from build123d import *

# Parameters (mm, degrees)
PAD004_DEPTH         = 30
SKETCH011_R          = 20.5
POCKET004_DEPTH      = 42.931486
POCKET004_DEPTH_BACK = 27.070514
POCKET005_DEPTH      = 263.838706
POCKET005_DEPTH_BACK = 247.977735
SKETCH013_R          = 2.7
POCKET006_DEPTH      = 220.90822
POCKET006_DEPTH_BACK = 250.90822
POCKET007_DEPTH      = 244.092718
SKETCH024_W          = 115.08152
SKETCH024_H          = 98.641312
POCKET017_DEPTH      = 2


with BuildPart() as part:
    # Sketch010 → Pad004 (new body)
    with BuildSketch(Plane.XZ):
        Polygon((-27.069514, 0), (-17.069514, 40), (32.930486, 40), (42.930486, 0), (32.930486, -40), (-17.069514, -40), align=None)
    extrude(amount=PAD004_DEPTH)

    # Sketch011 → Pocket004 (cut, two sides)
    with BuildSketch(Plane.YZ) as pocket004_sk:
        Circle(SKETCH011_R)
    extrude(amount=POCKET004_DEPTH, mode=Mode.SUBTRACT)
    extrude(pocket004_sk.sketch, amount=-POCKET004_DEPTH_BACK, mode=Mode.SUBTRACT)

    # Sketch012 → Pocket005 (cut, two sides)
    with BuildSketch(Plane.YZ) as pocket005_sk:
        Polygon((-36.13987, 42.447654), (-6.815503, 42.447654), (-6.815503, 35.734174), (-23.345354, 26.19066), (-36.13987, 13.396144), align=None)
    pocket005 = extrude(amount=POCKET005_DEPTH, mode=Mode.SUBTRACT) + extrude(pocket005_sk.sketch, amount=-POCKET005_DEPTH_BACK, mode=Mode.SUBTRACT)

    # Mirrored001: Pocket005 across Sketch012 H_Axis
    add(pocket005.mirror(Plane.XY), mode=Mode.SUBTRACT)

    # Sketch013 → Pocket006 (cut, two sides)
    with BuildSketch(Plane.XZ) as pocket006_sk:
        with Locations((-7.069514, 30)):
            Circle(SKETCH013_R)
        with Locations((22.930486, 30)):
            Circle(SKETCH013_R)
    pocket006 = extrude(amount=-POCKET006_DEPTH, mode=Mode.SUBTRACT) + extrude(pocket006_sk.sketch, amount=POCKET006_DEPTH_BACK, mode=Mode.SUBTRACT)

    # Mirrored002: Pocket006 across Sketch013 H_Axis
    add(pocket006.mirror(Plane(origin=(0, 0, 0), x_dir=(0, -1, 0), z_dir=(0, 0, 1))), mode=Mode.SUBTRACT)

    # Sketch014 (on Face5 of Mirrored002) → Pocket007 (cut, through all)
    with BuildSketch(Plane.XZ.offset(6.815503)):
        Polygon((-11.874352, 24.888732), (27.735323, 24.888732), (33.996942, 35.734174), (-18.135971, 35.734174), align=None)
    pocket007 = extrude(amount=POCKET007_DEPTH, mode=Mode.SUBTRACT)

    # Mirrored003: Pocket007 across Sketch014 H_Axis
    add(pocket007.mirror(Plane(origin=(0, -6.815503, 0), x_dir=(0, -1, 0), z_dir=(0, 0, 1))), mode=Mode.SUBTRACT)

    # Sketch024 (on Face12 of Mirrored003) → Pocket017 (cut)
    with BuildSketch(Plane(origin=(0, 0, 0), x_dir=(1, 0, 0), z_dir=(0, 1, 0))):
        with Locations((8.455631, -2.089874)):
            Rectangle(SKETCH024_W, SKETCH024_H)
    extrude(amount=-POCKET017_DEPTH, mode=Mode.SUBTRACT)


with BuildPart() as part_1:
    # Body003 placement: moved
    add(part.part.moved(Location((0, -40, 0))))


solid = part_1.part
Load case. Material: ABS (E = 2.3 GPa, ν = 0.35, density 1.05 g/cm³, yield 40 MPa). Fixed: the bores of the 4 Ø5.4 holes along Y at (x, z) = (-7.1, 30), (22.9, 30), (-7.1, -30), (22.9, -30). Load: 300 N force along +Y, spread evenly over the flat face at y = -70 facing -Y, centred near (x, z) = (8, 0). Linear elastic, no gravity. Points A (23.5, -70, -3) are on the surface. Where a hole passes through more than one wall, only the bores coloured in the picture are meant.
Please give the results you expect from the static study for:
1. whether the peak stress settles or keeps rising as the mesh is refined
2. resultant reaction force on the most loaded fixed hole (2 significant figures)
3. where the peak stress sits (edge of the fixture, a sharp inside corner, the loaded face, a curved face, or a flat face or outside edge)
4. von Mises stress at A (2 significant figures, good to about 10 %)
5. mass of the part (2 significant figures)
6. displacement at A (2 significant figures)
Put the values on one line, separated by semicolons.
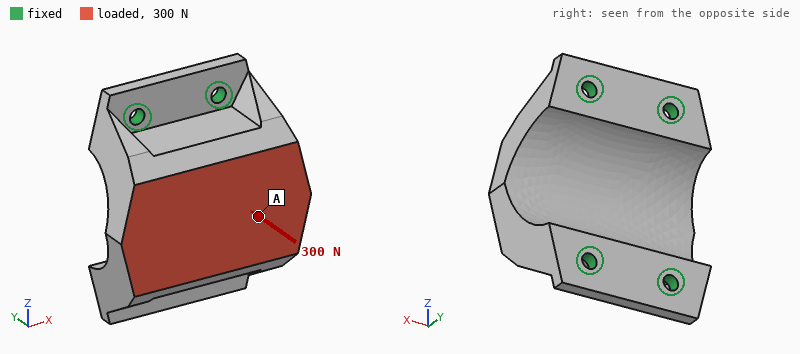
keeps rising; 92 N; edge of the fixture; 0.42 MPa; 62 g; 17 µm
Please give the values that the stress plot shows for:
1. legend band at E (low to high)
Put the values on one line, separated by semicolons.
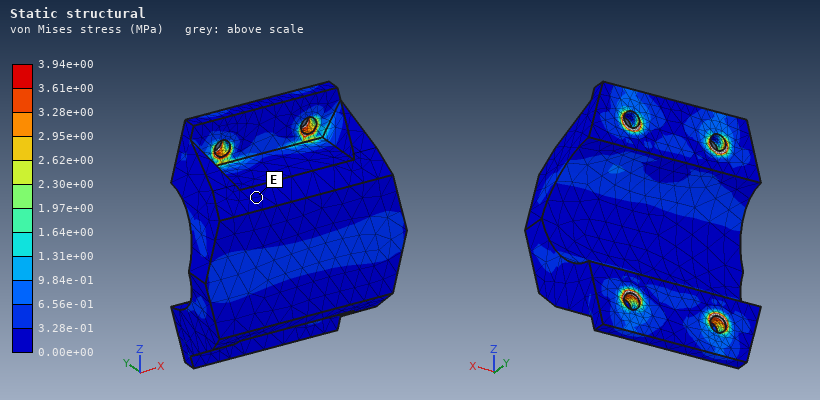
0.00e+00 to 3.28e-01 MPa
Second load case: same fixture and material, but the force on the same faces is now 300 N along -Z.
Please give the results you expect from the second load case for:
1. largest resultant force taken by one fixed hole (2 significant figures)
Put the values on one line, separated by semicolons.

100 N
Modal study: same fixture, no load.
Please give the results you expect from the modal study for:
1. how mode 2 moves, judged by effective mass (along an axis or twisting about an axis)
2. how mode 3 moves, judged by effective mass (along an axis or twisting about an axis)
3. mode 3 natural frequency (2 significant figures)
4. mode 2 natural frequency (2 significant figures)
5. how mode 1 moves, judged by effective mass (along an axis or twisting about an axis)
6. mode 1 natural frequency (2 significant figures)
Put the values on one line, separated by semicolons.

along Z; along Y; 3300 Hz; 3000 Hz; along X; 2000 Hz
